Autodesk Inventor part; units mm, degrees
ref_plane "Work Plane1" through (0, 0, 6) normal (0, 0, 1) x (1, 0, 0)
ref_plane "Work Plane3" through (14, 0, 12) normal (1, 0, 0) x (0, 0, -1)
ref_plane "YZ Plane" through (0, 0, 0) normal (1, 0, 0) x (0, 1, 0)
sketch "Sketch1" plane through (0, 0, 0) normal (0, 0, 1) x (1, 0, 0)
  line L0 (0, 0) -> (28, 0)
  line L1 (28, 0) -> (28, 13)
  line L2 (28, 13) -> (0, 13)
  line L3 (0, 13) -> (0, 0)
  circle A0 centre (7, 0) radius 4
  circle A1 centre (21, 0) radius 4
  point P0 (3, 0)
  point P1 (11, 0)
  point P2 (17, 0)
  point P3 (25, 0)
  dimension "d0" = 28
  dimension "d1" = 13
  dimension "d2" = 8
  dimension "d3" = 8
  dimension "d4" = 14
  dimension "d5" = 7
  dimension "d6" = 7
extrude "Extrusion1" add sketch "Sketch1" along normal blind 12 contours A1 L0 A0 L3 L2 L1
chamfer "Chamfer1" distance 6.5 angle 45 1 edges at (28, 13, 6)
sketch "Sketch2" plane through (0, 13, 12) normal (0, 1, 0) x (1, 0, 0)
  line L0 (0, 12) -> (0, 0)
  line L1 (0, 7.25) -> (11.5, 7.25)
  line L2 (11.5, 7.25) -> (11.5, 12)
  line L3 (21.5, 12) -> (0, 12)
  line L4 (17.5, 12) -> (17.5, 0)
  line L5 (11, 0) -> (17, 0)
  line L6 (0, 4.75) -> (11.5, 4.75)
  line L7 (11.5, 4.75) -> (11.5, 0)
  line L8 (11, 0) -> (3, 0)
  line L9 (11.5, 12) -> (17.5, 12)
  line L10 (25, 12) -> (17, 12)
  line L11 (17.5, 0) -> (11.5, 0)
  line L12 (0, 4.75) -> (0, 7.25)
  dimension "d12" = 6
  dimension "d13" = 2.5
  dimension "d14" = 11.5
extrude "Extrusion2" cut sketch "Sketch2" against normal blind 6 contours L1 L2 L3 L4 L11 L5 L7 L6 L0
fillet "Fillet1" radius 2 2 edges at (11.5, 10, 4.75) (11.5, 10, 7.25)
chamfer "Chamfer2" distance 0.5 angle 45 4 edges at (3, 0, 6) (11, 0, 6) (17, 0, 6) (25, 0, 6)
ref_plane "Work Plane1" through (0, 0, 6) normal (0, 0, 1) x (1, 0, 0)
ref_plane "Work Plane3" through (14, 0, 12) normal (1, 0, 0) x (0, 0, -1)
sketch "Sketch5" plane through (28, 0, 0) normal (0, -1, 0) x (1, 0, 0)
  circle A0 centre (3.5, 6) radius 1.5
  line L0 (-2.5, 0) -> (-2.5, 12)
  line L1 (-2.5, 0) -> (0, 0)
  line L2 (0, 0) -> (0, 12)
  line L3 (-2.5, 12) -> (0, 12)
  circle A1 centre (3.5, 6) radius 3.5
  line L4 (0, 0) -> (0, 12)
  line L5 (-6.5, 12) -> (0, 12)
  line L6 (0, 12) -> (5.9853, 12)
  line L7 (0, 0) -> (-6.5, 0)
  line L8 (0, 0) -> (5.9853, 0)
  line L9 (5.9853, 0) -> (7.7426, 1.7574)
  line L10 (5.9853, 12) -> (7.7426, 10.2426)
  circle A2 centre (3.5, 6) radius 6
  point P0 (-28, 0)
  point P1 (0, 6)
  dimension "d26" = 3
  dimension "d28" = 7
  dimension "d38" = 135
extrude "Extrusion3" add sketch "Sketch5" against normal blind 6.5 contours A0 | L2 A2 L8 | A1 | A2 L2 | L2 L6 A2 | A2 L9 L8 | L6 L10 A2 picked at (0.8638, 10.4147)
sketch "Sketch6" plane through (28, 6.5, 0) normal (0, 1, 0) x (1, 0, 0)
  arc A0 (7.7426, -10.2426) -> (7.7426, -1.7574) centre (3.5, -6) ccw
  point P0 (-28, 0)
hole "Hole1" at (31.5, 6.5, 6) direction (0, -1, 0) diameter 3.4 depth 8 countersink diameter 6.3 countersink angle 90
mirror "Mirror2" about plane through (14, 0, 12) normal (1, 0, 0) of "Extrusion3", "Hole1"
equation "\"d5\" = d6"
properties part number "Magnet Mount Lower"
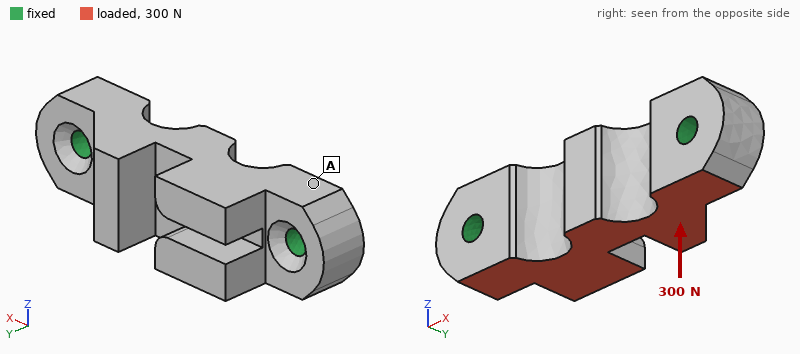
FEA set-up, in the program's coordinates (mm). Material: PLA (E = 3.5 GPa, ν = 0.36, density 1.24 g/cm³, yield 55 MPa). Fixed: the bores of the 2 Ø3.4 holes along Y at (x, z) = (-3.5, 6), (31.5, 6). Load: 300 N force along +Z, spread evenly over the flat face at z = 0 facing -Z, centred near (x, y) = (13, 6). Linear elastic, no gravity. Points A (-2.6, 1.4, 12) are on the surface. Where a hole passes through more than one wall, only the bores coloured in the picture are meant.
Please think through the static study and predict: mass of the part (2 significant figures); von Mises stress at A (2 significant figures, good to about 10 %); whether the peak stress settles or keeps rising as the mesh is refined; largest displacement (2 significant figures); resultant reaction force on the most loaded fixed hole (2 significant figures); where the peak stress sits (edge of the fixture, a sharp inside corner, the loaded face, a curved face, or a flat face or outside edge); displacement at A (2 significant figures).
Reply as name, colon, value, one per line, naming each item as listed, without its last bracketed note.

mass of the part: 5.0 g
von Mises stress at A: 3.1 MPa
whether the peak stress settles or keeps rising as the mesh is refined: keeps rising
largest displacement: 0.10 mm
resultant reaction force on the most loaded fixed hole: 160 N
where the peak stress sits: edge of the fixture
displacement at A: 0.016 mm
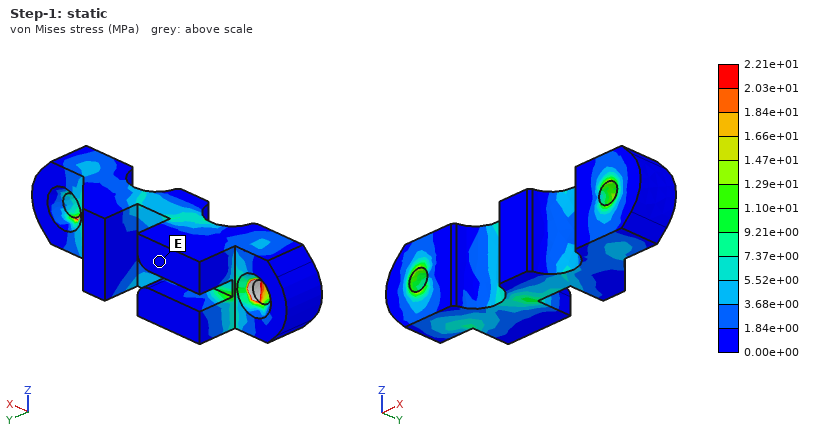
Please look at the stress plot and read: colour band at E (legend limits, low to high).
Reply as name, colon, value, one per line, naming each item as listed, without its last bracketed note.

colour band at E: 0.00e+00 to 1.84e+00 MPa
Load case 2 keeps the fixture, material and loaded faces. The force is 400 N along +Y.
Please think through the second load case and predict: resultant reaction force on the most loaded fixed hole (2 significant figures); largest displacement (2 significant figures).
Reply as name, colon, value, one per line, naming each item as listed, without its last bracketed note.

resultant reaction force on the most loaded fixed hole: 240 N
largest displacement: 0.22 mm
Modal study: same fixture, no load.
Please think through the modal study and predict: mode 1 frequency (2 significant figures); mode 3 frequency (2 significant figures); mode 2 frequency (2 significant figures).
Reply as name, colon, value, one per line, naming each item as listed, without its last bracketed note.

mode 1 frequency: 5500 Hz
mode 3 frequency: 7900 Hz
mode 2 frequency: 5600 Hz
